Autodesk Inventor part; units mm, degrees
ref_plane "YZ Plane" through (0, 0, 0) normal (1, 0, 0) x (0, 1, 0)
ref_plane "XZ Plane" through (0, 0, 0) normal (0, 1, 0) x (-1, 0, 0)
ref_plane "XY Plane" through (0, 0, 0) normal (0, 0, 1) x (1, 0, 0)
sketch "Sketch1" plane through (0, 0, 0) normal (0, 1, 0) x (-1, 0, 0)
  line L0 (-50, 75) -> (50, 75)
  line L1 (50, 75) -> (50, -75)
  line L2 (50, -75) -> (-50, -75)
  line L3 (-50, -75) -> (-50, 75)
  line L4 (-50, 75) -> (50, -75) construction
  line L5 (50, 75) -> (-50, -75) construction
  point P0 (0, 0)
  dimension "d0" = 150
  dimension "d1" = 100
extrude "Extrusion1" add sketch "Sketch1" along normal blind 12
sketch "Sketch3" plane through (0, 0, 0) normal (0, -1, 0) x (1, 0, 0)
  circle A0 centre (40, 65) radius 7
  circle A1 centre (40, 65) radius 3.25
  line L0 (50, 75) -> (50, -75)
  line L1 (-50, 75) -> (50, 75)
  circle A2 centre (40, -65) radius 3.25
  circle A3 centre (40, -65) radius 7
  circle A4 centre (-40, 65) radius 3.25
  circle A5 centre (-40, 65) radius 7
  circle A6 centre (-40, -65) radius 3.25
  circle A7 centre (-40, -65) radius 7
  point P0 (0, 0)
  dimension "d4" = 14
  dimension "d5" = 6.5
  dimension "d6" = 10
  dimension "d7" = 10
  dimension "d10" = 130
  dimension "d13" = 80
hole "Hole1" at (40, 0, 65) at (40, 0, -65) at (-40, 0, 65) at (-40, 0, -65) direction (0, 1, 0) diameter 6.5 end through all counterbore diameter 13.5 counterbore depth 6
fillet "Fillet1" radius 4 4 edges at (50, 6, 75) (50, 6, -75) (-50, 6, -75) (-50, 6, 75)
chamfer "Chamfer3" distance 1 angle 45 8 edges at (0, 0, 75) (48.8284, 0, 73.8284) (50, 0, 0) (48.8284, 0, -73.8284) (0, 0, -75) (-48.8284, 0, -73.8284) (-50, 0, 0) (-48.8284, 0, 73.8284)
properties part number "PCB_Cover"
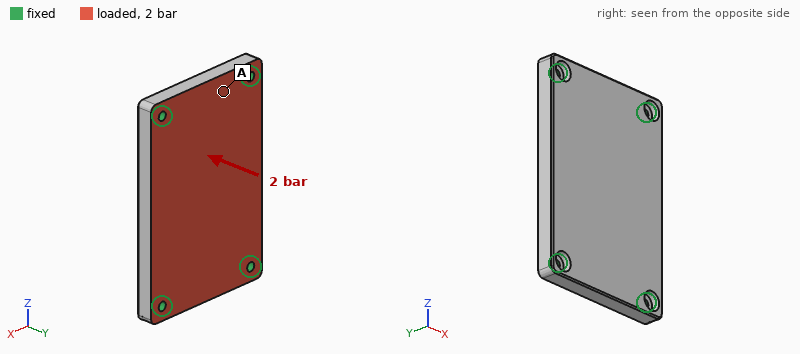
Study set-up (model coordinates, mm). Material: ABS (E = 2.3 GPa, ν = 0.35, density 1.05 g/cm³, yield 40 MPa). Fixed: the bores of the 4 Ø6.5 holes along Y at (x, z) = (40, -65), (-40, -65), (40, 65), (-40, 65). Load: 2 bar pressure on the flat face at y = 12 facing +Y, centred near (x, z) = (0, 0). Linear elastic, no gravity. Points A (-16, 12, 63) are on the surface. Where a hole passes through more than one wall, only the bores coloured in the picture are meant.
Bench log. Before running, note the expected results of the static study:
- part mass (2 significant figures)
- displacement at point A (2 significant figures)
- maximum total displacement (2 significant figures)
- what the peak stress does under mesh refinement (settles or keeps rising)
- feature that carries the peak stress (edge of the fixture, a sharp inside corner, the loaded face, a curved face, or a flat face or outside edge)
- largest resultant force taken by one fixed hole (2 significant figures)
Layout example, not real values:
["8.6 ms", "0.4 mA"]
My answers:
["180 g", "0.22 mm", "1.1 mm", "keeps rising", "edge of the fixture", "1.1 kN"]
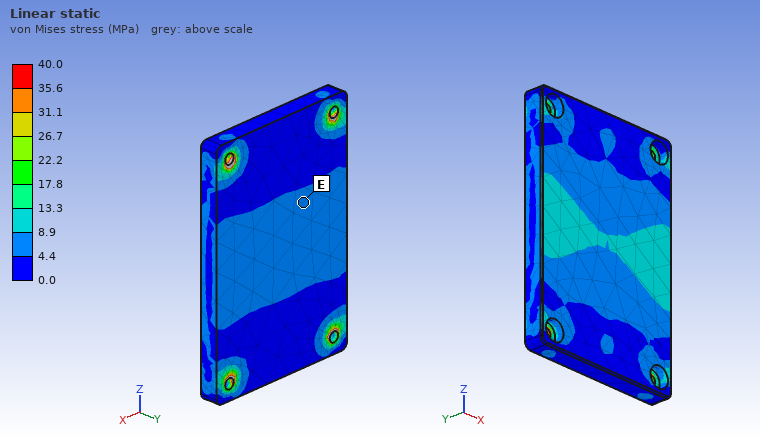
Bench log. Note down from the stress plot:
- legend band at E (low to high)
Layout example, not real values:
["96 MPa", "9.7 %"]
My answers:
["4.4 to 8.9 MPa"]
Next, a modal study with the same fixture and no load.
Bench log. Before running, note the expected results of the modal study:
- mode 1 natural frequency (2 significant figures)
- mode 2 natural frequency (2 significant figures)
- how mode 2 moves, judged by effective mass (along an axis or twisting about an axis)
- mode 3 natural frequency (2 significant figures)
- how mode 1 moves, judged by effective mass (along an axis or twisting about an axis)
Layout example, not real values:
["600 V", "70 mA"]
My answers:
["690 Hz", "1100 Hz", "twisting about Z", "1700 Hz", "along Y"]
